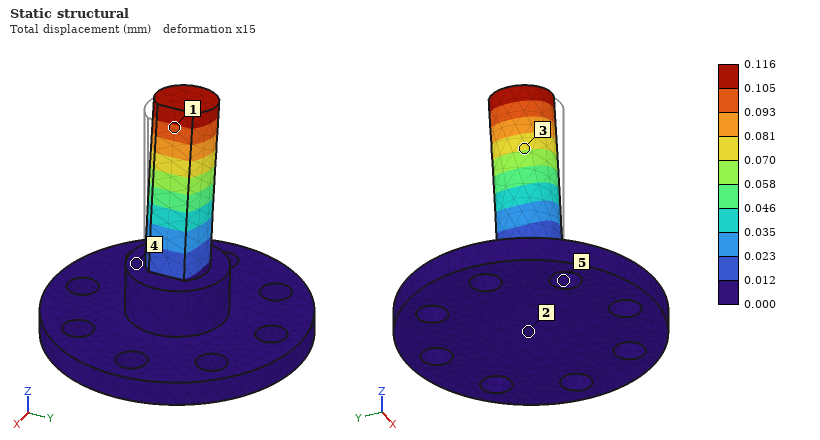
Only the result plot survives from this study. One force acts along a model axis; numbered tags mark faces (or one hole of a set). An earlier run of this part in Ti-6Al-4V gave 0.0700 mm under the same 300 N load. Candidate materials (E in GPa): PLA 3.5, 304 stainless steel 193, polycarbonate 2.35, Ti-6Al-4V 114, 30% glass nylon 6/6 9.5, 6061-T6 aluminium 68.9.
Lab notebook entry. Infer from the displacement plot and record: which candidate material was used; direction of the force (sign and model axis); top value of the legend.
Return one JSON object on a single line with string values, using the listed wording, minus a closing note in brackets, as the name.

{"which candidate material was used": "6061-T6 aluminium", "direction of the force": "-X", "top value of the legend": "0.116 mm"}
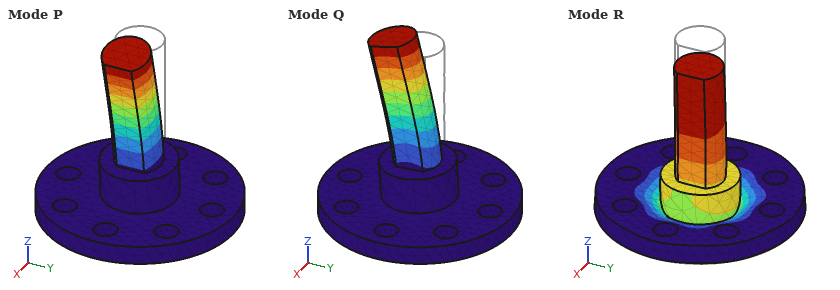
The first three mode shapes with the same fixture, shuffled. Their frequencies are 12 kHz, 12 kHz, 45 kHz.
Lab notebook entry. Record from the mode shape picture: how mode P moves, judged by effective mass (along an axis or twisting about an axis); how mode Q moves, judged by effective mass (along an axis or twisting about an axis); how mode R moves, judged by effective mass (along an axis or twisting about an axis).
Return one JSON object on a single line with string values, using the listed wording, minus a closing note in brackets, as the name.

{"how mode P moves, judged by effective mass": "along X", "how mode Q moves, judged by effective mass": "along Y", "how mode R moves, judged by effective mass": "along Z"}
